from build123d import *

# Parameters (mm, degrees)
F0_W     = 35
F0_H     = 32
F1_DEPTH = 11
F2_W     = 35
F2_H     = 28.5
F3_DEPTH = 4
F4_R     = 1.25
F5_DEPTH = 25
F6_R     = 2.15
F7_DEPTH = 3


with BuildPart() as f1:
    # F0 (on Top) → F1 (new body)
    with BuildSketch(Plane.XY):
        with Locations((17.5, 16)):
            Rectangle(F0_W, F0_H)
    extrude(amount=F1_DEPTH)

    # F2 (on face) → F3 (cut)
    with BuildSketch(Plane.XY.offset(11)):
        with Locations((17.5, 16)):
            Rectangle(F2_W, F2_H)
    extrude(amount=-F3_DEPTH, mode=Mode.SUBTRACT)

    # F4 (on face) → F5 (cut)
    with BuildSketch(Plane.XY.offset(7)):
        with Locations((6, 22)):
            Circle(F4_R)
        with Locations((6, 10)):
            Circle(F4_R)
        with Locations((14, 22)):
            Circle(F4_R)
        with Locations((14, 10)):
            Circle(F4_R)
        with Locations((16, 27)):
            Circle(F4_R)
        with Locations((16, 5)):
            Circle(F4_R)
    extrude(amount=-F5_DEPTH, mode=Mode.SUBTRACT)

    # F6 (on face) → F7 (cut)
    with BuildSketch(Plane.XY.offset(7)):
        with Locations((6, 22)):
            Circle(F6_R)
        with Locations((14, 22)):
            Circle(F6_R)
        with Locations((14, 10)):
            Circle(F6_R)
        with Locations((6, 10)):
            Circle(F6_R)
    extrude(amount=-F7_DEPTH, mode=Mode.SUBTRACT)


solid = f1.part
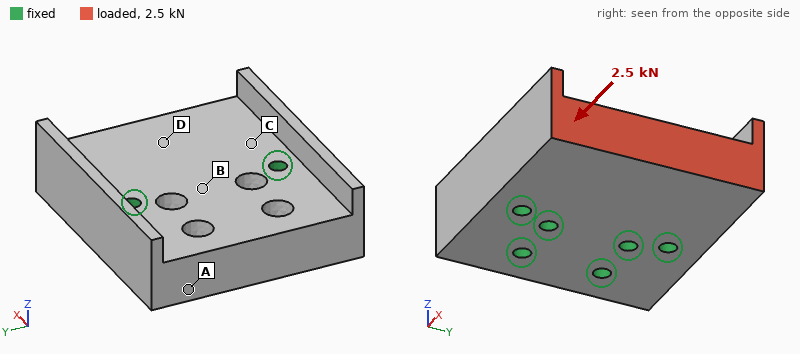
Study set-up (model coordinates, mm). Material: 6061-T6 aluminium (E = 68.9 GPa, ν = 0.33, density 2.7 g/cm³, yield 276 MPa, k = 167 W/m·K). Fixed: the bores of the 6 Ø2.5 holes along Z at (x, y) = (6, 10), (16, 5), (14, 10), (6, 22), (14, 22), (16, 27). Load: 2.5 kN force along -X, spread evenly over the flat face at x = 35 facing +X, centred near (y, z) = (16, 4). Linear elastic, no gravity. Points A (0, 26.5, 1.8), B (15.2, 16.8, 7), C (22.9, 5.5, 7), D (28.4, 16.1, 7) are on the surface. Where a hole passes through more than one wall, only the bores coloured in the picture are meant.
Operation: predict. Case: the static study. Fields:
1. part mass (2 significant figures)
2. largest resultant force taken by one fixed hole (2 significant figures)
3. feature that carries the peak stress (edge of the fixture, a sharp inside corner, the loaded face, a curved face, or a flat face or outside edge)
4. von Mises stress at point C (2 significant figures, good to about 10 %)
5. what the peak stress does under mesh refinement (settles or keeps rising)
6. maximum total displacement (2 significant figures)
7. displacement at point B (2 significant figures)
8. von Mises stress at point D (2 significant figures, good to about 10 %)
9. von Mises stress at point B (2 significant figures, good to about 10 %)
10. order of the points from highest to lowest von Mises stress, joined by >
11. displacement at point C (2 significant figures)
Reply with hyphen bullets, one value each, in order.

- 22 g
- 810 N
- edge of the fixture
- 13 MPa
- keeps rising
- 4.5 µm
- 0.98 µm
- 10 MPa
- 6.5 MPa
- C > D > B > A
- 1.8 µm
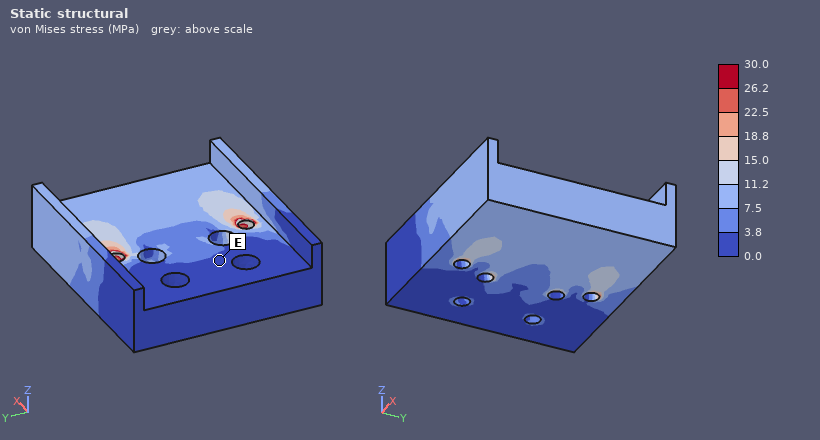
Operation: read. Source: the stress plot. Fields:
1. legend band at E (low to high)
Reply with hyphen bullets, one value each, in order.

- 0.0 to 3.8 MPa
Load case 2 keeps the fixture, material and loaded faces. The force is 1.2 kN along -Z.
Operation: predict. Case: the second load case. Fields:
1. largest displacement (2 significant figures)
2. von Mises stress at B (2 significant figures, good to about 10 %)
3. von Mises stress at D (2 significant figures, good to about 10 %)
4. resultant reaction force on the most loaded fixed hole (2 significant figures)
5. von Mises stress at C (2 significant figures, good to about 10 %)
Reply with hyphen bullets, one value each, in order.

- 51 µm
- 40 MPa
- 24 MPa
- 810 N
- 44 MPa
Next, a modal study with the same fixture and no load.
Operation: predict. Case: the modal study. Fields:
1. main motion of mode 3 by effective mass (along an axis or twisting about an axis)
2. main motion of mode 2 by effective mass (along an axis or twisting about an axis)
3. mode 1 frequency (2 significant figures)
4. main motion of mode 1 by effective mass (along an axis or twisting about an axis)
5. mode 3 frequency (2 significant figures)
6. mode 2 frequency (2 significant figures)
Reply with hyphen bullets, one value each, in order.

- along Y
- twisting about X
- 13 kHz
- along Z
- 29 kHz
- 21 kHz
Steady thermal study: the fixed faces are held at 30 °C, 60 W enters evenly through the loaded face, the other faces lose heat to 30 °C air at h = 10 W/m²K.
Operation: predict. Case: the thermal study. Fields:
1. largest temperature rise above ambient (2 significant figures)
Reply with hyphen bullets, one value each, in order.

- 31 K
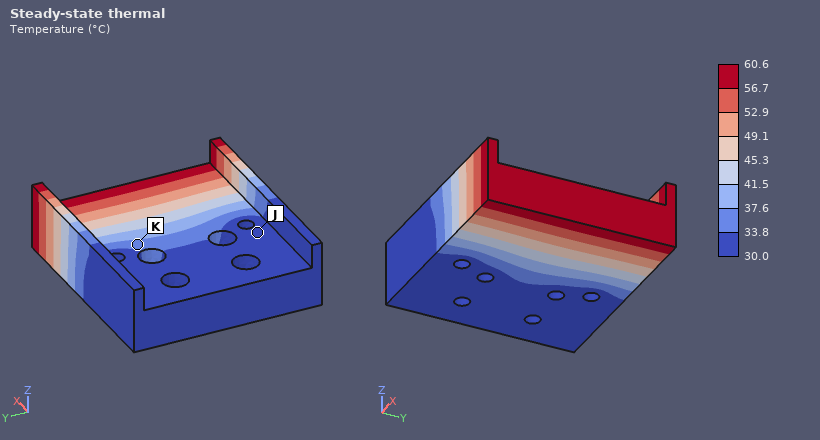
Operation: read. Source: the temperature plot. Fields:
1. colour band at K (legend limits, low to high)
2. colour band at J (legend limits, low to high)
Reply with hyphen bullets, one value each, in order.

- 33.8 to 37.6 °C
- 30.0 to 33.8 °C
